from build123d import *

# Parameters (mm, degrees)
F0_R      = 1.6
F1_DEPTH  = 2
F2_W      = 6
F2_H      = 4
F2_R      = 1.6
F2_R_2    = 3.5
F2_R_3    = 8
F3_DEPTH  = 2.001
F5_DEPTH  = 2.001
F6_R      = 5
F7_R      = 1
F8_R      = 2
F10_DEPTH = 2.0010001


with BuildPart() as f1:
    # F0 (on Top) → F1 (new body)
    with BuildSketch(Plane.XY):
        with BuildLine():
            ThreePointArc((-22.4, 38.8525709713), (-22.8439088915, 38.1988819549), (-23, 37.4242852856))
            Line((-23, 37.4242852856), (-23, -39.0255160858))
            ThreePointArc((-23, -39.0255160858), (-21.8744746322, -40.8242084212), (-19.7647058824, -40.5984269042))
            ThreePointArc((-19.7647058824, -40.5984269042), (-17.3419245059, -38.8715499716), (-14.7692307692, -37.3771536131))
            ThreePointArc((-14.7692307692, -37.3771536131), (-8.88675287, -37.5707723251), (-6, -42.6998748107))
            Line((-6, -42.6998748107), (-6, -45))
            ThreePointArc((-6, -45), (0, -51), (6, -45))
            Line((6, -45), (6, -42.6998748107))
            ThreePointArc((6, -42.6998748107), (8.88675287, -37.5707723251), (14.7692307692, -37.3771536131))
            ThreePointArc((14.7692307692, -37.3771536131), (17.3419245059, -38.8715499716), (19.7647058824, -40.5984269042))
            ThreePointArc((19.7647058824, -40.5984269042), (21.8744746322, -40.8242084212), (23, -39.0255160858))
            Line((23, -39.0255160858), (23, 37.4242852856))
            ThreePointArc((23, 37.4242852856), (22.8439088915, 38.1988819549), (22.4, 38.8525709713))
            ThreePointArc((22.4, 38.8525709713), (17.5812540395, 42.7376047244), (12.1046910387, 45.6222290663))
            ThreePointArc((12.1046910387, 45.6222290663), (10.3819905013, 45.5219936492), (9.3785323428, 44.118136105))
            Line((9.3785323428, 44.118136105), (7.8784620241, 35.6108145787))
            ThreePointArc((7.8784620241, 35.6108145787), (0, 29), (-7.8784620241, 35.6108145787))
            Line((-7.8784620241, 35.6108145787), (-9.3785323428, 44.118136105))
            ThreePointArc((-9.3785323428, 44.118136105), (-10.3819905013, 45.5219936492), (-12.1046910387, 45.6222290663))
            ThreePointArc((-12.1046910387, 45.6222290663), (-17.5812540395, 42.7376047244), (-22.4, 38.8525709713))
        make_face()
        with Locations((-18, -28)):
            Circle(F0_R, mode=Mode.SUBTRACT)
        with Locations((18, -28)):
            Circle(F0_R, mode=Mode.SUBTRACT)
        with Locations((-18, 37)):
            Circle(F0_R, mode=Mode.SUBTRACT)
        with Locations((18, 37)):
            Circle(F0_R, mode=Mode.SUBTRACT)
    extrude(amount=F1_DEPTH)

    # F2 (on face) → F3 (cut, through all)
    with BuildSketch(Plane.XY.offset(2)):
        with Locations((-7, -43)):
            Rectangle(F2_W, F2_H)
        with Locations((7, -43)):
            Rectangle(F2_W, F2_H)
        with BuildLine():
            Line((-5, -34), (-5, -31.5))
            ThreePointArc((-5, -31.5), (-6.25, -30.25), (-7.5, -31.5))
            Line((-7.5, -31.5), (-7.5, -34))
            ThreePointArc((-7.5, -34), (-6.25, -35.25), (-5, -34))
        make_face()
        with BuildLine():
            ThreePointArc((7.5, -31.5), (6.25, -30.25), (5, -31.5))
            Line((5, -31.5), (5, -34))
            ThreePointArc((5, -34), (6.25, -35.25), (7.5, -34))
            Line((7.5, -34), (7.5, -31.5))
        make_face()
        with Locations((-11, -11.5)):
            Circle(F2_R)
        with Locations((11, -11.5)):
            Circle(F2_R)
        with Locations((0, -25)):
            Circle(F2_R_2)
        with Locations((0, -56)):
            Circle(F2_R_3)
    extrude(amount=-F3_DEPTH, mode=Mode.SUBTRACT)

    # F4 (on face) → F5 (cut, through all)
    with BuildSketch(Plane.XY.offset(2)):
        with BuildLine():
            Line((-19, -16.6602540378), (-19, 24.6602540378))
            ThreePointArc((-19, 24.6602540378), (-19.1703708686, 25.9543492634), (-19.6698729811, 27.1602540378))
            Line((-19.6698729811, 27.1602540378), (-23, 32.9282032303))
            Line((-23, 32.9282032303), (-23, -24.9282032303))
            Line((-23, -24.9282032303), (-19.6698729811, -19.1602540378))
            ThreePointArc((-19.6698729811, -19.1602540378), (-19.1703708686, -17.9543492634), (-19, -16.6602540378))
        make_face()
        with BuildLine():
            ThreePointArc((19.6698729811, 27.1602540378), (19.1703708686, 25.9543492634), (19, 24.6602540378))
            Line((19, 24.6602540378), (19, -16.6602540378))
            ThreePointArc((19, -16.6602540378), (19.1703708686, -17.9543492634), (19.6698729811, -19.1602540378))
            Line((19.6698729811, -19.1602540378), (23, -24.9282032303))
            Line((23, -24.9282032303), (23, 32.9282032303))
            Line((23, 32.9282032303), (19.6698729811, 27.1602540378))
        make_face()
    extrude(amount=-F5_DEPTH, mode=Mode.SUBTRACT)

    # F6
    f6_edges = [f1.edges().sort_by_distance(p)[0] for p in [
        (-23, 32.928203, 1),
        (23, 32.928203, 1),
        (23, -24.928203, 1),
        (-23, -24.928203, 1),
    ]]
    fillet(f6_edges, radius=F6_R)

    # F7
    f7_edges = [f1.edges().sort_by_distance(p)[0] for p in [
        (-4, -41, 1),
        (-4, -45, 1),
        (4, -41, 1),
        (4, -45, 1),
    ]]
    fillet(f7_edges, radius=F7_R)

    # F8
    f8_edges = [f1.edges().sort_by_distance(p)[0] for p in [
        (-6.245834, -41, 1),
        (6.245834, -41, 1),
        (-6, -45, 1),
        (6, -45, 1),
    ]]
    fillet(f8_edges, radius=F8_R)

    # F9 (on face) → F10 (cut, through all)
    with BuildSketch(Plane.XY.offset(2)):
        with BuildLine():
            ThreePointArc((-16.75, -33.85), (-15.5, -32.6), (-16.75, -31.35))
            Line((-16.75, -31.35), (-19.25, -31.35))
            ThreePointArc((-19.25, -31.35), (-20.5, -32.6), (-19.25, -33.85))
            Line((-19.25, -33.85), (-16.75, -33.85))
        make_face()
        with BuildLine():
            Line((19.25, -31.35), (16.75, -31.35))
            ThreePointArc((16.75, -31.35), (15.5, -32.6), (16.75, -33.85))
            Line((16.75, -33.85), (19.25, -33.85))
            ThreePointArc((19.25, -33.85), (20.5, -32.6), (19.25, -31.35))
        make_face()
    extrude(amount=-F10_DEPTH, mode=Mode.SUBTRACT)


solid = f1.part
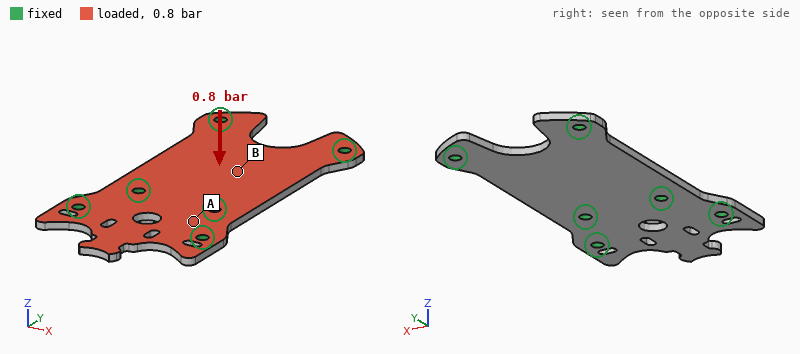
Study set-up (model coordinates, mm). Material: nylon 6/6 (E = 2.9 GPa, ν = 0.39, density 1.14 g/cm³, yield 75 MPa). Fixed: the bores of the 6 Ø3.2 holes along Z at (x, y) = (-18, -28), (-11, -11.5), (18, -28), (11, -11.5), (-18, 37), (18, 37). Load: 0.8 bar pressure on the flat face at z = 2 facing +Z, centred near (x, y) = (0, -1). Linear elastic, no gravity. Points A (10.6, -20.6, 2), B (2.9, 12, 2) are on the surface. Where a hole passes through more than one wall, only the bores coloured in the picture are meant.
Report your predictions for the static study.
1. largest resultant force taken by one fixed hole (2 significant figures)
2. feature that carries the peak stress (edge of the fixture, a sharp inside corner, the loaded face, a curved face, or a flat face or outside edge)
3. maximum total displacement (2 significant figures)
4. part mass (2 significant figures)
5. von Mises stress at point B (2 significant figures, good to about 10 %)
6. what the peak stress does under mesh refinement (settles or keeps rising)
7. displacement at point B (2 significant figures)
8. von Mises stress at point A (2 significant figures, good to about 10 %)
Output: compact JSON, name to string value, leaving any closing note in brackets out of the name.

{"largest resultant force taken by one fixed hole": "52 N", "feature that carries the peak stress": "edge of the fixture", "maximum total displacement": "1.1 mm", "part mass": "7.1 g", "von Mises stress at point B": "10 MPa", "what the peak stress does under mesh refinement": "keeps rising", "displacement at point B": "0.64 mm", "von Mises stress at point A": "3.6 MPa"}
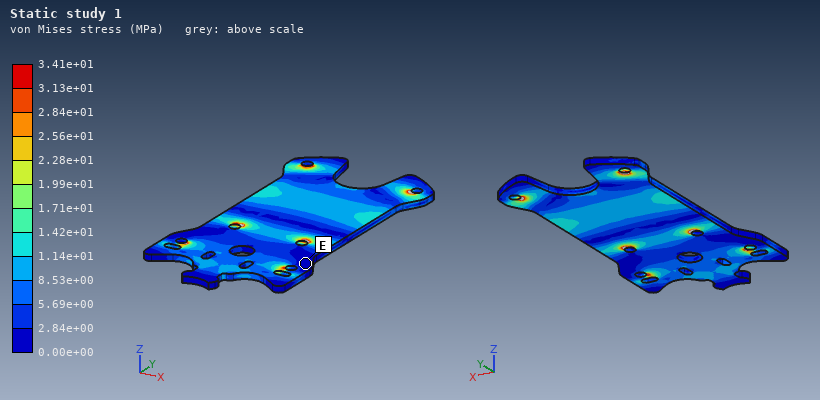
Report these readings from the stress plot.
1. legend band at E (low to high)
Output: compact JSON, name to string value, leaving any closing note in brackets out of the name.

{"legend band at E": "0.00e+00 to 2.84e+00 MPa"}
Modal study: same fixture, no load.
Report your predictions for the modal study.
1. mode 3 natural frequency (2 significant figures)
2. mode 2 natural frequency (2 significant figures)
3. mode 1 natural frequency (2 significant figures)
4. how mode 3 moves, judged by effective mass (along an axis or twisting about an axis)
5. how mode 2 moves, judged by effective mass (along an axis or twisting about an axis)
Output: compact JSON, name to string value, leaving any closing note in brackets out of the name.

{"mode 3 natural frequency": "1900 Hz", "mode 2 natural frequency": "1300 Hz", "mode 1 natural frequency": "1300 Hz", "how mode 3 moves, judged by effective mass": "twisting about Y", "how mode 2 moves, judged by effective mass": "along Z"}
